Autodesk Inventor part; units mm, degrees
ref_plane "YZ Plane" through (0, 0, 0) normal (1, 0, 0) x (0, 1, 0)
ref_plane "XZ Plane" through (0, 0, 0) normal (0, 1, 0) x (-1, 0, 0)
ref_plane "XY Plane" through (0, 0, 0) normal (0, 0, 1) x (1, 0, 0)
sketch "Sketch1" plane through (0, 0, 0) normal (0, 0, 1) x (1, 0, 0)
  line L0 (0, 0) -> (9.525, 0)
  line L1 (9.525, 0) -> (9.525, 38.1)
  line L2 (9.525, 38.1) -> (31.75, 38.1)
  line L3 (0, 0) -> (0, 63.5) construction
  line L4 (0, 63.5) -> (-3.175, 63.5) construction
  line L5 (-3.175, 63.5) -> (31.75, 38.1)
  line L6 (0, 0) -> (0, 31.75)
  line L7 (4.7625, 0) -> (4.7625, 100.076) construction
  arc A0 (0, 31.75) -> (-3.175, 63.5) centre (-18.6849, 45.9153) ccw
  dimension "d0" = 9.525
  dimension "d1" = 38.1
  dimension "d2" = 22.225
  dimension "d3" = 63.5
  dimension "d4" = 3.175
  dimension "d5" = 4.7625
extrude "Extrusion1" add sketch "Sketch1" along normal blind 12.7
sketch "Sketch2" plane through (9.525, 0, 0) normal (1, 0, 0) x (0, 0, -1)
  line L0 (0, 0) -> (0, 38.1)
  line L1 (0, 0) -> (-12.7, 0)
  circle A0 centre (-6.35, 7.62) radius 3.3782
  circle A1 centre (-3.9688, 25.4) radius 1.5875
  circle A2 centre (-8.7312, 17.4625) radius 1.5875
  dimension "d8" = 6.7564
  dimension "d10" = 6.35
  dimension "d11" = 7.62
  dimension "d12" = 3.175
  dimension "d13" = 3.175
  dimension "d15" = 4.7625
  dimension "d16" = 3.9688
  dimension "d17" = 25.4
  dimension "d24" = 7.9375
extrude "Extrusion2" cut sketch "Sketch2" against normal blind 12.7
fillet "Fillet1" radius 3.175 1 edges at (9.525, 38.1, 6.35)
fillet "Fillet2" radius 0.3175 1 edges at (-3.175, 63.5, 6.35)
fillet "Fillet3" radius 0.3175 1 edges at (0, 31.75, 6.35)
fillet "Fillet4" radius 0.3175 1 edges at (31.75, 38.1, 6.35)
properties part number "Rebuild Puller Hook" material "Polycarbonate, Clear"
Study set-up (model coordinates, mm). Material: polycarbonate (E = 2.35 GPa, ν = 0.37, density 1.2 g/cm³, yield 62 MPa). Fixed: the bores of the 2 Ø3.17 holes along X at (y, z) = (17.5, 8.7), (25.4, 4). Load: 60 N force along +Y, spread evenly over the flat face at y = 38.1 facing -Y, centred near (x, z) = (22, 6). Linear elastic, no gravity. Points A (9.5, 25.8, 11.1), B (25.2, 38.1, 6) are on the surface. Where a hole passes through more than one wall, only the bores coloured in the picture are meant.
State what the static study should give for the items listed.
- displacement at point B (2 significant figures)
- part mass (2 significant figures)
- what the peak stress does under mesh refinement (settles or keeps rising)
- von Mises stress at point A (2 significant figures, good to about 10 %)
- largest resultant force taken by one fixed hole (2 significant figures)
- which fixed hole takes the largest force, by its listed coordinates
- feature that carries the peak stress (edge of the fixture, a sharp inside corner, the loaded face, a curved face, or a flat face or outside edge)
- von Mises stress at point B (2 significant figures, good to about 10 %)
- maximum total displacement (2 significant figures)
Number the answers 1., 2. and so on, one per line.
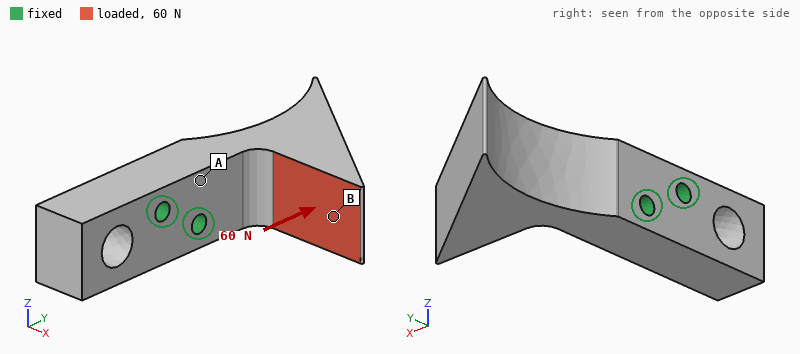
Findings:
1. 0.28 mm
2. 9.2 g
3. keeps rising
4. 3.6 MPa
5. 48 N
6. (25.4, 4)
7. edge of the fixture
8. 1.3 MPa
9. 0.38 mm
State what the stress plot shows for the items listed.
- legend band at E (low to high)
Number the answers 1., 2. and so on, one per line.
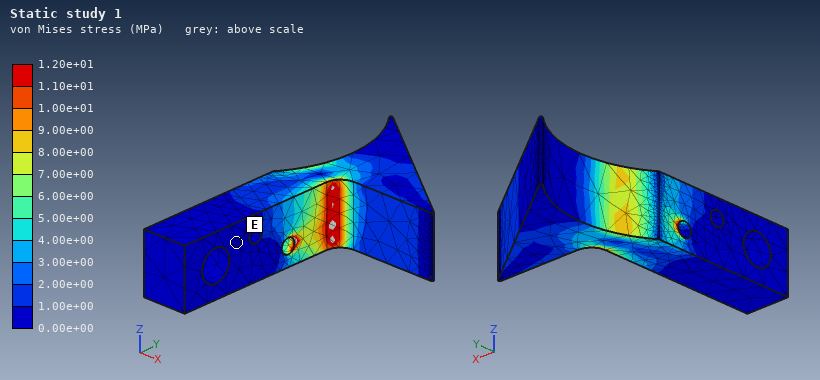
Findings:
1. 0.00e+00 to 1.00e+00 MPa
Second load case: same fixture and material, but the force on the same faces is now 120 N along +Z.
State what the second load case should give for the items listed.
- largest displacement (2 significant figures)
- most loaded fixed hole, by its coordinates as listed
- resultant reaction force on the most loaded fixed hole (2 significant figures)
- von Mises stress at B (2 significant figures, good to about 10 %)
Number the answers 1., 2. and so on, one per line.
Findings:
1. 0.73 mm
2. (25.4, 4)
3. 210 N
4. 2.7 MPa
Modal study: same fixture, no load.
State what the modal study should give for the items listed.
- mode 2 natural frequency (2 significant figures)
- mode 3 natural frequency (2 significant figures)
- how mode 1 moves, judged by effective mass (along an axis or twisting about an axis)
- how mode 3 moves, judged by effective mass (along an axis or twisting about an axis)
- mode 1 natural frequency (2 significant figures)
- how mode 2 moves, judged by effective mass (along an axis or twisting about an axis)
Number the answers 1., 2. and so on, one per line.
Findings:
1. 1700 Hz
2. 2400 Hz
3. along X
4. twisting about Y
5. 1300 Hz
6. along Z
